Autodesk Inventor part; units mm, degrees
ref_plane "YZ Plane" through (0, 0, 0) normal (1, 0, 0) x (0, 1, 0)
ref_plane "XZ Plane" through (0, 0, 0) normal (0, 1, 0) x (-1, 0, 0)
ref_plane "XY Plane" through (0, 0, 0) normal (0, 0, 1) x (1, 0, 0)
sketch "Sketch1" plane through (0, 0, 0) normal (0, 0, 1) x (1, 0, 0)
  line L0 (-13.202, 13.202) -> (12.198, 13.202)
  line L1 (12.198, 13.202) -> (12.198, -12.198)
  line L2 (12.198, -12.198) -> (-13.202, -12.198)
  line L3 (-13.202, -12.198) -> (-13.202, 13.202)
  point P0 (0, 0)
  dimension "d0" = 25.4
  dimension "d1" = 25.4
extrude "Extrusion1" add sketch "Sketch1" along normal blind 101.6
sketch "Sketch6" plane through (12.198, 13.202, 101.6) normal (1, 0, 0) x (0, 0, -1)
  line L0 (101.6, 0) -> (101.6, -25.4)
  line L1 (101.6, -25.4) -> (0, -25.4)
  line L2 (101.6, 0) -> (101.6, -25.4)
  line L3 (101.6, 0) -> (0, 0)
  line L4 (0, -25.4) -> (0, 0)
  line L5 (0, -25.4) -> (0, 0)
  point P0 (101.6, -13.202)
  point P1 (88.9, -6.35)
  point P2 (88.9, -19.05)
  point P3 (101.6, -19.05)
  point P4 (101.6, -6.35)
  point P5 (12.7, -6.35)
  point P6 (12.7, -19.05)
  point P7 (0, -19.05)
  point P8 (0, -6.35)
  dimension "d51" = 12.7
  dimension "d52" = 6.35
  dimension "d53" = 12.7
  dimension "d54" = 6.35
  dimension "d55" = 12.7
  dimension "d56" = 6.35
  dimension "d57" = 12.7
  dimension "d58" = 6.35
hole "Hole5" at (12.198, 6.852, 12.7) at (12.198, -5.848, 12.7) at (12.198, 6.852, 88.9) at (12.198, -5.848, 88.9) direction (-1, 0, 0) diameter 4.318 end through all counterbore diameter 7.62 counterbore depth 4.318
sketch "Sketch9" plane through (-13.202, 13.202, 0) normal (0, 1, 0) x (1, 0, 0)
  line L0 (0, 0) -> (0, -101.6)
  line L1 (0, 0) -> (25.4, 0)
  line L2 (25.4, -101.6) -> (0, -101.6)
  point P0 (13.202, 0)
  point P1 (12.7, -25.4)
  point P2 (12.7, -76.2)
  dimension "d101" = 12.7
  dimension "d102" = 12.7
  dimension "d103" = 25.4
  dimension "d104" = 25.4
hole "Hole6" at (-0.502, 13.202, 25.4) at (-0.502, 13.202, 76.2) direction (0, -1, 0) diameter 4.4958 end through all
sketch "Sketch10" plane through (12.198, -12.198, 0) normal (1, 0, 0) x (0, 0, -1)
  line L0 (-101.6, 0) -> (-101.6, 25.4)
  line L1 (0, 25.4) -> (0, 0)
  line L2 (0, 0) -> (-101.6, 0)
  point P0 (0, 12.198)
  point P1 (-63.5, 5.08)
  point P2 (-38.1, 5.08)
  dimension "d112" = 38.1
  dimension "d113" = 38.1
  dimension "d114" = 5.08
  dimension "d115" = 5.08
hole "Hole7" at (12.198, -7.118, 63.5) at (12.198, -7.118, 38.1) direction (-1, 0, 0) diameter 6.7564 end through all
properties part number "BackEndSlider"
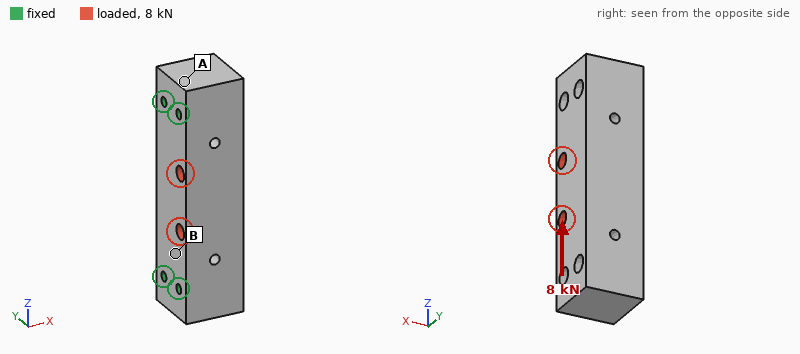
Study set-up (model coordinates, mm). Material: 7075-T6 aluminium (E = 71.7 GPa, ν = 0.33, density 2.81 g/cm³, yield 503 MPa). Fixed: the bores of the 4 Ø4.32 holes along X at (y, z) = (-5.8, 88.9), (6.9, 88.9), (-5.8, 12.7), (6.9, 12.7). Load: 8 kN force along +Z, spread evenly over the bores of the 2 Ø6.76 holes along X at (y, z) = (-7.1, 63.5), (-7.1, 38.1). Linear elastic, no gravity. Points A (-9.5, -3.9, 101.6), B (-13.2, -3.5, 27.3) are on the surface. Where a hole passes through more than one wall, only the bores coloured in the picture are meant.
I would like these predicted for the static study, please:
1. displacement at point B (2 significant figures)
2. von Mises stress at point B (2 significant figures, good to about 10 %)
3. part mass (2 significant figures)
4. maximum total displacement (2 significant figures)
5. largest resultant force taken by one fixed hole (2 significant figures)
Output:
1.6 µm
7.8 MPa
170 g
4.7 µm
2.1 kN
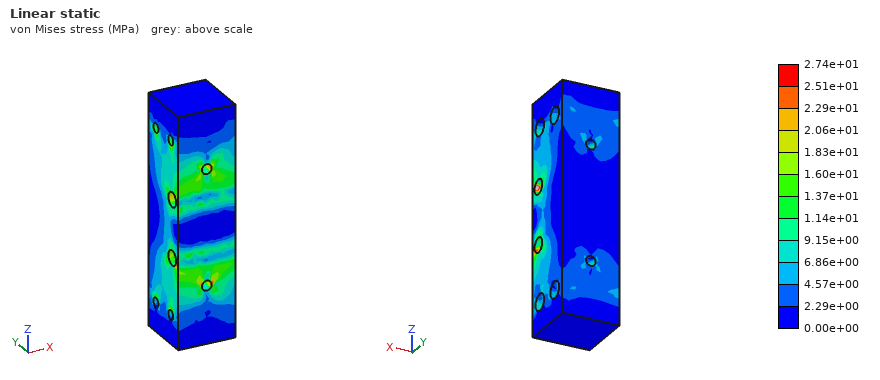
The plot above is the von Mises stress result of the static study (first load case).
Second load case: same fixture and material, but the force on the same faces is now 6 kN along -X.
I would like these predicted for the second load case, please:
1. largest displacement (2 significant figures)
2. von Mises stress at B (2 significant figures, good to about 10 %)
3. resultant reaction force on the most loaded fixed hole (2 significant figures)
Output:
19 µm
15 MPa
2.3 kN
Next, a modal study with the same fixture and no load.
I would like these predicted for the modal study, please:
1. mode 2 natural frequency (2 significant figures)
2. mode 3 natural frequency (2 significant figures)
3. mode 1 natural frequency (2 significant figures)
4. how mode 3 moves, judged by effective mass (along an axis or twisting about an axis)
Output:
14 kHz
18 kHz
13 kHz
twisting about Z
